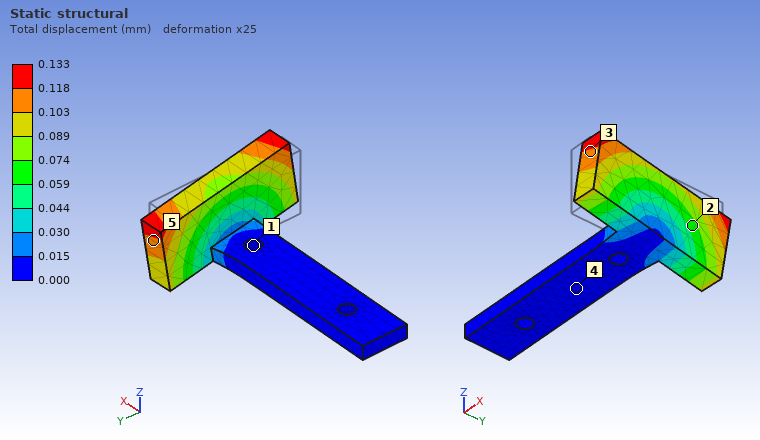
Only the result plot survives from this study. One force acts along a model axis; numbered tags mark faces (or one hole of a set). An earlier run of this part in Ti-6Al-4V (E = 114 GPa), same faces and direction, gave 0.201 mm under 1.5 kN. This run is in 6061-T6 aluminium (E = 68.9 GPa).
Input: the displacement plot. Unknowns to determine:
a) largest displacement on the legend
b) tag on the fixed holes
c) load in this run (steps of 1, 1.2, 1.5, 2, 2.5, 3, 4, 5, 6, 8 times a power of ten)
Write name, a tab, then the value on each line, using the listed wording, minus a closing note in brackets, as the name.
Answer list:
largest displacement on the legend	0.133 mm
tag on the fixed holes	1
load in this run	600 N
